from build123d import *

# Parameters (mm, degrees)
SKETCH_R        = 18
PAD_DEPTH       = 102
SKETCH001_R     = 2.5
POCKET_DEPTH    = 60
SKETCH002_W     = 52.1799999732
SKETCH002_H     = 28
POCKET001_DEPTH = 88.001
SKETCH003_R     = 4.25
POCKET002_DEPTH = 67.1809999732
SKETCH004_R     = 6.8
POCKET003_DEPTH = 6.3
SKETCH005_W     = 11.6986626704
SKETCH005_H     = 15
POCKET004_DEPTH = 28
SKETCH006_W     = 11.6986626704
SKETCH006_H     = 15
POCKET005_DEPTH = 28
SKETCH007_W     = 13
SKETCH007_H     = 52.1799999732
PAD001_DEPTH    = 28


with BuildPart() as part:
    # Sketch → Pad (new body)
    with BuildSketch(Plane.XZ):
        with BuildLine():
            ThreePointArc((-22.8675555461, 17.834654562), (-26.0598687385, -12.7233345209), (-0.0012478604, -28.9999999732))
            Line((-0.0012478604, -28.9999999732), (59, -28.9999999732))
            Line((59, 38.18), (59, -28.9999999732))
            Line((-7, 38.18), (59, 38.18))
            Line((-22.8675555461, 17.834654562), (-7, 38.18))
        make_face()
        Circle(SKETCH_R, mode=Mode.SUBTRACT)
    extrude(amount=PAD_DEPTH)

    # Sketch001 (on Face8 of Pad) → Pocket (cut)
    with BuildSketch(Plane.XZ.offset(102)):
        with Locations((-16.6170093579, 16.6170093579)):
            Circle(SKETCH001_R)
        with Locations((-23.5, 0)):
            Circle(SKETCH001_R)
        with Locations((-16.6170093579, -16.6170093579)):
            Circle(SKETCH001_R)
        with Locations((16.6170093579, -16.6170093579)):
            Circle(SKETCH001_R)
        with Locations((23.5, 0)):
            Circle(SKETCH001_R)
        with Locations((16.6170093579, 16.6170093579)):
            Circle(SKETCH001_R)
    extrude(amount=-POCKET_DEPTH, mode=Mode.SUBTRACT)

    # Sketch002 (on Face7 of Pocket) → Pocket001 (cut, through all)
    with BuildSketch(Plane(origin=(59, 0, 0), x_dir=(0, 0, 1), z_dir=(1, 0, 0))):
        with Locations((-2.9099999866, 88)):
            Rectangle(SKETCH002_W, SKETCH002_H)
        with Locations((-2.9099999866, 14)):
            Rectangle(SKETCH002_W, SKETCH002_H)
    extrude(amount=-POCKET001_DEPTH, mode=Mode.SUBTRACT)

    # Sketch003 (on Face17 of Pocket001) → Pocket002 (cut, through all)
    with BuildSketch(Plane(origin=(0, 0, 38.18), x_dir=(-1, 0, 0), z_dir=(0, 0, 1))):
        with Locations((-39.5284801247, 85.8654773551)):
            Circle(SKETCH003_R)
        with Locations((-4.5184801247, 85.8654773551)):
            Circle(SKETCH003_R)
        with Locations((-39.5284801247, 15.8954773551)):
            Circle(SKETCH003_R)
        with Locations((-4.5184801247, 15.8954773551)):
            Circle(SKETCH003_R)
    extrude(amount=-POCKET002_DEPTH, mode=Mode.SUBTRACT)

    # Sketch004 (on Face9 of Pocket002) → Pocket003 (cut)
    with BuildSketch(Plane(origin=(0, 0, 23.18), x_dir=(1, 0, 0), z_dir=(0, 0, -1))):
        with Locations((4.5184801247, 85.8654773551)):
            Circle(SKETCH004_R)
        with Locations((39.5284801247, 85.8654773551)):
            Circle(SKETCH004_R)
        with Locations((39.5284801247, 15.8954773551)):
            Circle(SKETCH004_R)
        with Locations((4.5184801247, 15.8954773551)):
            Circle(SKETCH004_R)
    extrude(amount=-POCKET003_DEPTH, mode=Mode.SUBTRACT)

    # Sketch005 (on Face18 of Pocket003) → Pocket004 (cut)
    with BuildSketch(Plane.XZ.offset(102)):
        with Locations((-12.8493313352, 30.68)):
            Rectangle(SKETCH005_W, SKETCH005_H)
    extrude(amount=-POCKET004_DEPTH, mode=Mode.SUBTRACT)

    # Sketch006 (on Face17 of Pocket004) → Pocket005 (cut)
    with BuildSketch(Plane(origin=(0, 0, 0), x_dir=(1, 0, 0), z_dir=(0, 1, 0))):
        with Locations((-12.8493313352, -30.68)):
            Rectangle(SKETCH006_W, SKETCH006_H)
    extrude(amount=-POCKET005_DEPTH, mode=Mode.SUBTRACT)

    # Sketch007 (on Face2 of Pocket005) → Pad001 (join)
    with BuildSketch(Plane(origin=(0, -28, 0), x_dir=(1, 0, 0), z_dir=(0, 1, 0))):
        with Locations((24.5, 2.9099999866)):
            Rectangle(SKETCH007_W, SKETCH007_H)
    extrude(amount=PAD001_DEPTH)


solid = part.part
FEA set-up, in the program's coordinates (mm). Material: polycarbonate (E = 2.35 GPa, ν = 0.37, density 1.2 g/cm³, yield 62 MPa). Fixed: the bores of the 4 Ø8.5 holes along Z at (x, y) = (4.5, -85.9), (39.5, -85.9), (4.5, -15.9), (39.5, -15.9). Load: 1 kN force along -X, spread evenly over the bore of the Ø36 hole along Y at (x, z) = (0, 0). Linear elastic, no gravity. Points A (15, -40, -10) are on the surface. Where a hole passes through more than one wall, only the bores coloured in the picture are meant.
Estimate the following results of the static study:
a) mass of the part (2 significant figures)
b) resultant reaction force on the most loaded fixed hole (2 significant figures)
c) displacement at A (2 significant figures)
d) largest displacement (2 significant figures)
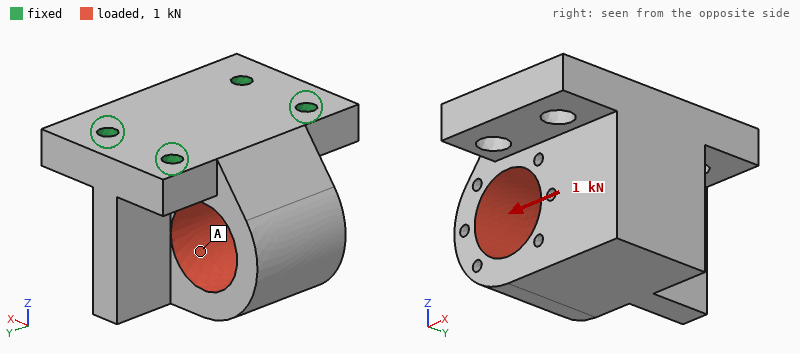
320 g
610 N
0.12 mm
0.19 mm
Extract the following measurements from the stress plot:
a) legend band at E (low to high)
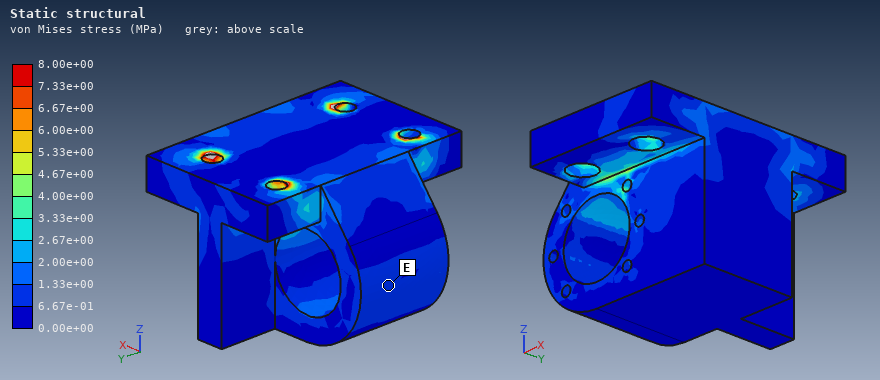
6.67e-01 to 1.33e+00 MPa
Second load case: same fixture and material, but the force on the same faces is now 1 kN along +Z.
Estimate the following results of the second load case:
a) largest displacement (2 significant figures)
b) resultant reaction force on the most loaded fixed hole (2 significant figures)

0.16 mm
620 N
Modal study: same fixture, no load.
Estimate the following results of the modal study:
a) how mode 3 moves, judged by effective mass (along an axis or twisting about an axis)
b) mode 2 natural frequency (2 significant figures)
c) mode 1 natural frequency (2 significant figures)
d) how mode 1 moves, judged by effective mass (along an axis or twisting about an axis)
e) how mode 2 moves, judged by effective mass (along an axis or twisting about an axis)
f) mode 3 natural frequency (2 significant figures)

along Z
1500 Hz
870 Hz
along X
along Y
2000 Hz
